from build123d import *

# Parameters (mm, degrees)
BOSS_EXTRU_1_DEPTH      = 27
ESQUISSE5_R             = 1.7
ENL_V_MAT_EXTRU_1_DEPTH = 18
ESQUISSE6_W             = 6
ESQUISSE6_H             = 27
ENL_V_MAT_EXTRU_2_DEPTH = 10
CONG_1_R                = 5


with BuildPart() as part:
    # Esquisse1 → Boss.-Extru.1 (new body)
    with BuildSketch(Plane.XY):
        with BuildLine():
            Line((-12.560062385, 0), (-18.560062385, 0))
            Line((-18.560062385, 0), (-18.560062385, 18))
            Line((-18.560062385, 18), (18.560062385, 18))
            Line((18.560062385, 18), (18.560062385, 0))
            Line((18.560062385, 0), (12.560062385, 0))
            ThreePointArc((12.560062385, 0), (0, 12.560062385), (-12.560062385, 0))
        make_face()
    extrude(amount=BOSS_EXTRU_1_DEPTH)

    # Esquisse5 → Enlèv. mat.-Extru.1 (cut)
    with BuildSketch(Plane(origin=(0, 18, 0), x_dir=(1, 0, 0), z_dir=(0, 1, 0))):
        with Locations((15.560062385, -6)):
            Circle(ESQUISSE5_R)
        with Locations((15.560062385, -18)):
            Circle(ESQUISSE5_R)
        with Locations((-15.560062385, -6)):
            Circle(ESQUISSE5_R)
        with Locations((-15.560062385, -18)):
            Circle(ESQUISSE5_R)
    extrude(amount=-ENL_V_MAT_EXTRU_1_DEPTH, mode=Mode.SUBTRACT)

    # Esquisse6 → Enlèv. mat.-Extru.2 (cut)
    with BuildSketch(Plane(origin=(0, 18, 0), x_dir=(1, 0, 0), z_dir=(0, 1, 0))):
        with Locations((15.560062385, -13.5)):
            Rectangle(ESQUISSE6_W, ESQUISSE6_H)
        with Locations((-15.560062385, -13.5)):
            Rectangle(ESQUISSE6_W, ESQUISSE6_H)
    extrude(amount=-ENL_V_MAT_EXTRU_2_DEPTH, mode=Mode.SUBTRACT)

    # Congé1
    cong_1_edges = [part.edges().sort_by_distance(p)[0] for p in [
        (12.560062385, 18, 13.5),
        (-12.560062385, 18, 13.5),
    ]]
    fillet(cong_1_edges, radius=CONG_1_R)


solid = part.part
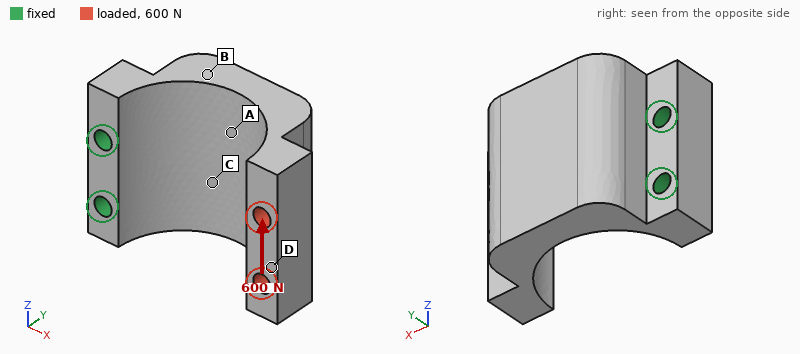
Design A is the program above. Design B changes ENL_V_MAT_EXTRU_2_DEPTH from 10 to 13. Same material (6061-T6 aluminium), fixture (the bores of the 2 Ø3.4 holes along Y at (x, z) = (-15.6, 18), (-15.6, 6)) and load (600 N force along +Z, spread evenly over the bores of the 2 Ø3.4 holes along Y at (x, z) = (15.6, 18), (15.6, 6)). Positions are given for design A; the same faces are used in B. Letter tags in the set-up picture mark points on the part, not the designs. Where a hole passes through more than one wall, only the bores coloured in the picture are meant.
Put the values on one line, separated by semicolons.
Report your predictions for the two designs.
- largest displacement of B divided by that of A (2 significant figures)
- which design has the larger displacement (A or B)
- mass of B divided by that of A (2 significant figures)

2.2; B; 0.89
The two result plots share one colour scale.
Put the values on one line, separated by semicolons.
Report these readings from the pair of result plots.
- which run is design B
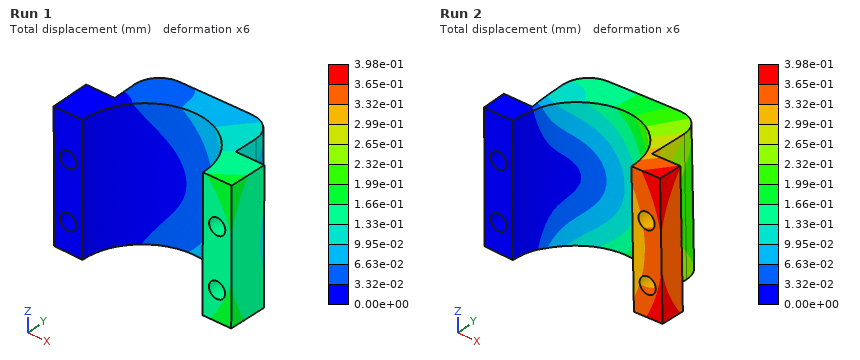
Run 2
